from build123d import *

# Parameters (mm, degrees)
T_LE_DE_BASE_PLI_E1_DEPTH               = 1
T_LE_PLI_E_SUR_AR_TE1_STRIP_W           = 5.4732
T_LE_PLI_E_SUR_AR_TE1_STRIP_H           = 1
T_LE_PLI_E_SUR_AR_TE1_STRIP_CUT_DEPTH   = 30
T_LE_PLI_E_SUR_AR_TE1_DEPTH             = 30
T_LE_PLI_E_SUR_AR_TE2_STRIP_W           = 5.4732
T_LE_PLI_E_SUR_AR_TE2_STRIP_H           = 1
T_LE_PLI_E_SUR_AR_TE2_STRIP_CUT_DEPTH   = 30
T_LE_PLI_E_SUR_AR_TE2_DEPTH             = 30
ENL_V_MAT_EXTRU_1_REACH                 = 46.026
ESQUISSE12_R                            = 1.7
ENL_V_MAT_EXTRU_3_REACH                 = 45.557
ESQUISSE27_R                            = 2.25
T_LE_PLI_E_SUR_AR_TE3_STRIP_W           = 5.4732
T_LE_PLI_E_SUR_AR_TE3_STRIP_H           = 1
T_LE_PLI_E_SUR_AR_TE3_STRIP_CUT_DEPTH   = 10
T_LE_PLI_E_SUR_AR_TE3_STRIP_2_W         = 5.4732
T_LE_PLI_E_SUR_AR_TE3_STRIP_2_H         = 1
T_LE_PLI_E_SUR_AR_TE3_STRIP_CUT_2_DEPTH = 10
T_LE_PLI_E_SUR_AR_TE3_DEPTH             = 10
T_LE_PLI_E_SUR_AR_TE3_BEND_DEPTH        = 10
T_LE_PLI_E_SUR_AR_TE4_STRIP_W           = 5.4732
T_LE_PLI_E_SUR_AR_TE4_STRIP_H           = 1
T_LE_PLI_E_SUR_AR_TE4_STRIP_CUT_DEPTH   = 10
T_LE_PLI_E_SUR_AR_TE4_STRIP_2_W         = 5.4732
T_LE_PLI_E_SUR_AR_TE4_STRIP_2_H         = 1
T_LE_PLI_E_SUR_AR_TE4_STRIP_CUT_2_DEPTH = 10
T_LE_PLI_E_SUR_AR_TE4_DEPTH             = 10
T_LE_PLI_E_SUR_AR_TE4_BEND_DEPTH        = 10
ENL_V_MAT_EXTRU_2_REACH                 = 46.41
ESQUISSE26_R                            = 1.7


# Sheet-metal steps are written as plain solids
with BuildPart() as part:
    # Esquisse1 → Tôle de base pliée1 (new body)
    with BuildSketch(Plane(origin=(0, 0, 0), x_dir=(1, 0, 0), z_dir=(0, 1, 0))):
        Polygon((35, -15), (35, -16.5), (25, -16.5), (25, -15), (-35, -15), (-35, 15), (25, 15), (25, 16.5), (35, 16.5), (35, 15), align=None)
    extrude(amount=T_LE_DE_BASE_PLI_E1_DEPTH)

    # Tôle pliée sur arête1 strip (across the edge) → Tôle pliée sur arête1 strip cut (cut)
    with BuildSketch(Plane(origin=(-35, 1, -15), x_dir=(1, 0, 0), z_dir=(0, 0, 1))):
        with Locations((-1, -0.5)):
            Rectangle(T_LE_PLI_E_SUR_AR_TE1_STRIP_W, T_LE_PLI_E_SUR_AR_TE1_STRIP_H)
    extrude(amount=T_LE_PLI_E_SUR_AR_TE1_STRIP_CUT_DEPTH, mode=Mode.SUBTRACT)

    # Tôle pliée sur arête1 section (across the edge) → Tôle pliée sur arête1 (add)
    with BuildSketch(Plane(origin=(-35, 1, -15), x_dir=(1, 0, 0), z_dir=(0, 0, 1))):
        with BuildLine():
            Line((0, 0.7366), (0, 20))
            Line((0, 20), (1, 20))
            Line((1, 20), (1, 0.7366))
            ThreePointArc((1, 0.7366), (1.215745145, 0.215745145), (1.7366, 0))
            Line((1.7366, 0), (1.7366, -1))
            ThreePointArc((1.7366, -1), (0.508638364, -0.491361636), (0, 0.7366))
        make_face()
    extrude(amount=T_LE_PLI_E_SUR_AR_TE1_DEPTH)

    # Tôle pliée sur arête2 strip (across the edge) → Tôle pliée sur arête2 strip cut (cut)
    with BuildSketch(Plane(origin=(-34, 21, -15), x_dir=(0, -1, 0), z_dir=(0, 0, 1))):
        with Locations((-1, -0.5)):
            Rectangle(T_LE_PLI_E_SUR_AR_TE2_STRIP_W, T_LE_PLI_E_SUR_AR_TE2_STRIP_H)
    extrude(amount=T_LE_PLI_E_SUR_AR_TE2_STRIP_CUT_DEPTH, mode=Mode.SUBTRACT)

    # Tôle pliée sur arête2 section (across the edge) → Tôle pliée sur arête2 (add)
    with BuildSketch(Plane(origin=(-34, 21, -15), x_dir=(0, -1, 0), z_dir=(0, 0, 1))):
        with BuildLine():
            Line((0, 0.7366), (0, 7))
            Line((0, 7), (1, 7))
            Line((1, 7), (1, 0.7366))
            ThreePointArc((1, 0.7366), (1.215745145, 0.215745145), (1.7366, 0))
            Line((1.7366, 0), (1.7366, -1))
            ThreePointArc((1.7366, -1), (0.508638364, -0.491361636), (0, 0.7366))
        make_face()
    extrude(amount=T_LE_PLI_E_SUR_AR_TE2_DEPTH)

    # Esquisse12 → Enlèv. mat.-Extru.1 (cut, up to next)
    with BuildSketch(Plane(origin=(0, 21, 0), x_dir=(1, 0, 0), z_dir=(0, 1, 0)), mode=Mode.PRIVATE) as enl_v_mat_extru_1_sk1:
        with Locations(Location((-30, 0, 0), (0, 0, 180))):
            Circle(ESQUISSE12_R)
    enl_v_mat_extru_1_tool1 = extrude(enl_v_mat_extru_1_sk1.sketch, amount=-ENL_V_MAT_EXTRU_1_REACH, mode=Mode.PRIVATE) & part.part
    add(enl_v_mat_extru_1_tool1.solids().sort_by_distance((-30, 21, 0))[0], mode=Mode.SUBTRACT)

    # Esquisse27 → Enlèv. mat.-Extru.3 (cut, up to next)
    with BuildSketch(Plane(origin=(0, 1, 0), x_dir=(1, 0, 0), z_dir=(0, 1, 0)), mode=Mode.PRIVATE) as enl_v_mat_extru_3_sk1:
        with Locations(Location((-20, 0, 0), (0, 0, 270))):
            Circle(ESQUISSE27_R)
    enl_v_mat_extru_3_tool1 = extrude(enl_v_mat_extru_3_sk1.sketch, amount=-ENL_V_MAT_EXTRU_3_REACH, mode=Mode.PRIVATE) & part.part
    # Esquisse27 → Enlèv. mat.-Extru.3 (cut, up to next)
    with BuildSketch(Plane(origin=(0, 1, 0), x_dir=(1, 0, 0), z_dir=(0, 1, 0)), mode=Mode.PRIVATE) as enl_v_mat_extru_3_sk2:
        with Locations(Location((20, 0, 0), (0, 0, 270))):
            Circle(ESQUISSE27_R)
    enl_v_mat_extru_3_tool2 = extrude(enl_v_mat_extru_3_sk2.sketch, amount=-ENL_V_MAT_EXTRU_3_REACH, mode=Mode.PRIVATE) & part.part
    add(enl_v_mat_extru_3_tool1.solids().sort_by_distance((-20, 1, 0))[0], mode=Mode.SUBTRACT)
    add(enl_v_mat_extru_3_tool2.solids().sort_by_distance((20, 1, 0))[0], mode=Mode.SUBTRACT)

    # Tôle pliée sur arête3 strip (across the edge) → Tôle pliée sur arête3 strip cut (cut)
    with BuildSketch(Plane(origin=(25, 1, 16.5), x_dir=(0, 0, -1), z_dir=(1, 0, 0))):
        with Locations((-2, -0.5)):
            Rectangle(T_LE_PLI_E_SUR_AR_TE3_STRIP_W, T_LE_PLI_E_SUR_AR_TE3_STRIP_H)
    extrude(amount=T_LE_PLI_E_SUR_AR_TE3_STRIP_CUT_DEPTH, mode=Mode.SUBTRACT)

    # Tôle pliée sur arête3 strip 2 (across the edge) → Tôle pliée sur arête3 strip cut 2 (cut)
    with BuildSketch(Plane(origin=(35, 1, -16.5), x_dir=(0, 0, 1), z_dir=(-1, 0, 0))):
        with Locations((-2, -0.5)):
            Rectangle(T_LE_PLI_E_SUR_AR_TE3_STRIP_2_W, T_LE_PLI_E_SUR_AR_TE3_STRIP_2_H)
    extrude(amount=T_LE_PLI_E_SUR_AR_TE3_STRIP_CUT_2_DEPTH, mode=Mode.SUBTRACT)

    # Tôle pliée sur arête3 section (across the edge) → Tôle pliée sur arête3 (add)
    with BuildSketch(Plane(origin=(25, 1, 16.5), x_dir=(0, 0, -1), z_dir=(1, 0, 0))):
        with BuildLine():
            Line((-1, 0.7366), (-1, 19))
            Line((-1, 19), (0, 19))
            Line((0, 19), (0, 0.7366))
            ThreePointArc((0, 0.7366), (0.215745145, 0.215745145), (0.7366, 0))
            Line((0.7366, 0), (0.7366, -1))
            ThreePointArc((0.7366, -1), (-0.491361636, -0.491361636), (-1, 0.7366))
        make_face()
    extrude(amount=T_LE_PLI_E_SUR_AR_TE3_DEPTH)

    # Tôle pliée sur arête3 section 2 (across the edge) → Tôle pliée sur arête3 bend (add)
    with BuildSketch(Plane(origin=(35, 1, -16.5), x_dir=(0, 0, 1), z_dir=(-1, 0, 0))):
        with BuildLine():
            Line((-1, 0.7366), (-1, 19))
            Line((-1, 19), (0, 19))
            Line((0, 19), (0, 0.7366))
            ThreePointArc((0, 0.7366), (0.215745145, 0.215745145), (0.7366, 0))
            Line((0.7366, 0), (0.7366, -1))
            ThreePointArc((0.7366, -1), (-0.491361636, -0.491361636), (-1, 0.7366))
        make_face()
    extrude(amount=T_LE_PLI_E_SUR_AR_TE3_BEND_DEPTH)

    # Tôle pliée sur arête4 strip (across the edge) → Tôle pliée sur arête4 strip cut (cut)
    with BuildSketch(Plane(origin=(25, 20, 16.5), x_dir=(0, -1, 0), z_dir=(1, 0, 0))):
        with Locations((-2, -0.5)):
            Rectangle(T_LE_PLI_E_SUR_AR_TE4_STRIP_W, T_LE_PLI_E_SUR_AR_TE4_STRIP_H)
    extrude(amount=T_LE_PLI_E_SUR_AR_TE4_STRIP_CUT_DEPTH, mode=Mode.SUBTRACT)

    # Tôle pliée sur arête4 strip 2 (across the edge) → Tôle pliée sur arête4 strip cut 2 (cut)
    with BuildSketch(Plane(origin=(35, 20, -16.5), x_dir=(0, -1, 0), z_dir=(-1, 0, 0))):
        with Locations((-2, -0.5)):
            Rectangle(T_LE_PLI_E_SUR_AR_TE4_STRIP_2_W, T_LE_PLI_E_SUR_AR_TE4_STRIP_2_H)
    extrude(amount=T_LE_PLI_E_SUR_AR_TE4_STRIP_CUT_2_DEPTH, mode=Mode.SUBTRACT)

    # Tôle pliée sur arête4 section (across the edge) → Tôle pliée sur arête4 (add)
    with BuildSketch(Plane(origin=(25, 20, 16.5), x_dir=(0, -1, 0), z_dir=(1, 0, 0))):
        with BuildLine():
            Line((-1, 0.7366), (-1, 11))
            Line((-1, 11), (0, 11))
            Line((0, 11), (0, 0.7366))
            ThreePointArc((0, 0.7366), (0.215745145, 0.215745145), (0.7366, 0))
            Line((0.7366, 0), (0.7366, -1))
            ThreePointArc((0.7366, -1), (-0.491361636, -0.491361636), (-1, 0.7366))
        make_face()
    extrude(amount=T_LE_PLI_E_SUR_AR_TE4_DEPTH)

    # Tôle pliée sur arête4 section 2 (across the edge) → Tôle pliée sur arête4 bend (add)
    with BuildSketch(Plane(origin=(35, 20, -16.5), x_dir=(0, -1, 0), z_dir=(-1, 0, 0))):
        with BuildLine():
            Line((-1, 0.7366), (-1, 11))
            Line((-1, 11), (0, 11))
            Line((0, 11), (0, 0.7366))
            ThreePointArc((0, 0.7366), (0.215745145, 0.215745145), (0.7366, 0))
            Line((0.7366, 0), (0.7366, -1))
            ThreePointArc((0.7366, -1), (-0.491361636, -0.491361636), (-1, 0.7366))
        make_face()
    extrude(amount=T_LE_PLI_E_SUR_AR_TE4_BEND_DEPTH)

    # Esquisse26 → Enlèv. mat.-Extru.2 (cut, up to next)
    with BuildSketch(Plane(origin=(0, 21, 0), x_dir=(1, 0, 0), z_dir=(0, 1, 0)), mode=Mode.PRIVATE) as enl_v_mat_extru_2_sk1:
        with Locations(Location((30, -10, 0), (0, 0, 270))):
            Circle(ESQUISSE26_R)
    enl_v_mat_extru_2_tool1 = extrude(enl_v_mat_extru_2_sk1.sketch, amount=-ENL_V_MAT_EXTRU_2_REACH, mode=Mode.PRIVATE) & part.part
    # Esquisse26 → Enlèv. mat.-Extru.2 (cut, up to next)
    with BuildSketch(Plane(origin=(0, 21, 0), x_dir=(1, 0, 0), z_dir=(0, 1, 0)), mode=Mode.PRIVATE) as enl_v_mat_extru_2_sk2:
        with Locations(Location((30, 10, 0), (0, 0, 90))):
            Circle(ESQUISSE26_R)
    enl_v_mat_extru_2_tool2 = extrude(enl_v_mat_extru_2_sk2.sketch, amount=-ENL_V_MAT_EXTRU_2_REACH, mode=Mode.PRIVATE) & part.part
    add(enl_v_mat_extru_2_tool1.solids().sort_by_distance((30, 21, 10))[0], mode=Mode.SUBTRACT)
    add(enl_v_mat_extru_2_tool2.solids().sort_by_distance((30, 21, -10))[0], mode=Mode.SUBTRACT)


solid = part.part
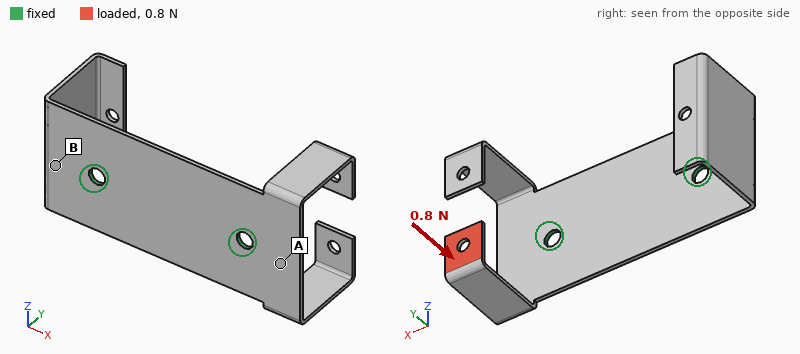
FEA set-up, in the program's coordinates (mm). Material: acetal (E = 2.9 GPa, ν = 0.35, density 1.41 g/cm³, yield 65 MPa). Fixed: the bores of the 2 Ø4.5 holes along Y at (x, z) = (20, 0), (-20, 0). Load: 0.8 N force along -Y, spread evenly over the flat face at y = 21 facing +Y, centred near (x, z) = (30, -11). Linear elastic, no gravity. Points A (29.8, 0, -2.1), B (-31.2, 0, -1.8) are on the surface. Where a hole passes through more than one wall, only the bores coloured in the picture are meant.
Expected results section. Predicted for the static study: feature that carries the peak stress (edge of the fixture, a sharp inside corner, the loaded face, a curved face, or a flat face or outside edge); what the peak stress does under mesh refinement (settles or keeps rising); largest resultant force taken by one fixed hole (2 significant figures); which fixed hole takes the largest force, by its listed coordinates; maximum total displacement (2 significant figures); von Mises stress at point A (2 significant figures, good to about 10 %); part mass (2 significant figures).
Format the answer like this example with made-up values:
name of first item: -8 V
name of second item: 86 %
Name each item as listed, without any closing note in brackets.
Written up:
feature that carries the peak stress: edge of the fixture
what the peak stress does under mesh refinement: keeps rising
largest resultant force taken by one fixed hole: 0.84 N
which fixed hole takes the largest force, by its listed coordinates: (20, 0)
maximum total displacement: 0.80 mm
von Mises stress at point A: 1.4 MPa
part mass: 4.9 g
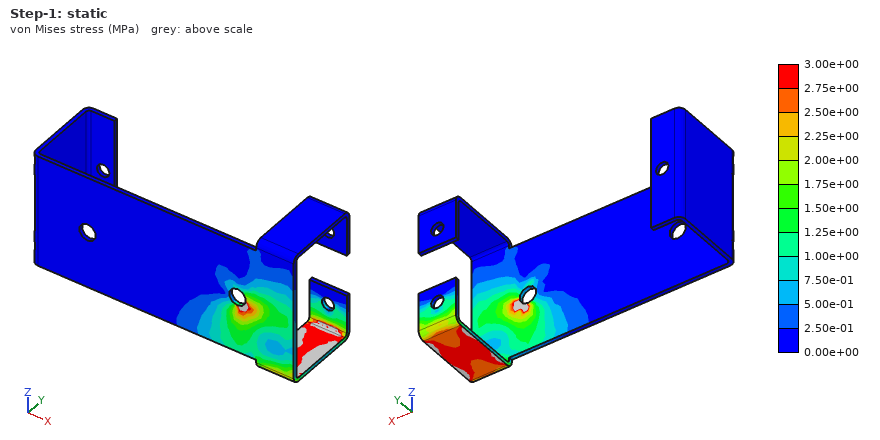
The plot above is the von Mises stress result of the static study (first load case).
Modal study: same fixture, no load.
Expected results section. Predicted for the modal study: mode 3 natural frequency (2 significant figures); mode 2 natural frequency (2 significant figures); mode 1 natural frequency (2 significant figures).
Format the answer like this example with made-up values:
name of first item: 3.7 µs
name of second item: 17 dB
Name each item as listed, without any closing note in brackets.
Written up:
mode 3 natural frequency: 200 Hz
mode 2 natural frequency: 200 Hz
mode 1 natural frequency: 190 Hz
